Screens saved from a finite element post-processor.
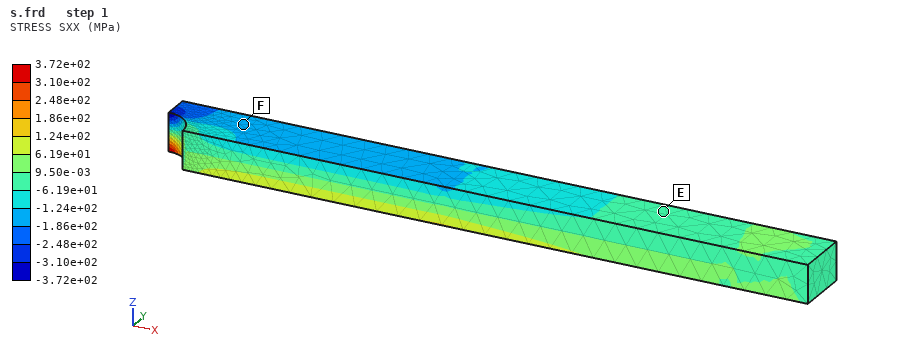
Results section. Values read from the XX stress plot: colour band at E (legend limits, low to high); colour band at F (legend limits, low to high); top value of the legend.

-6.19e+01 to 9.50e-03 MPa
-1.86e+02 to -1.24e+02 MPa
3.72e+02 MPa
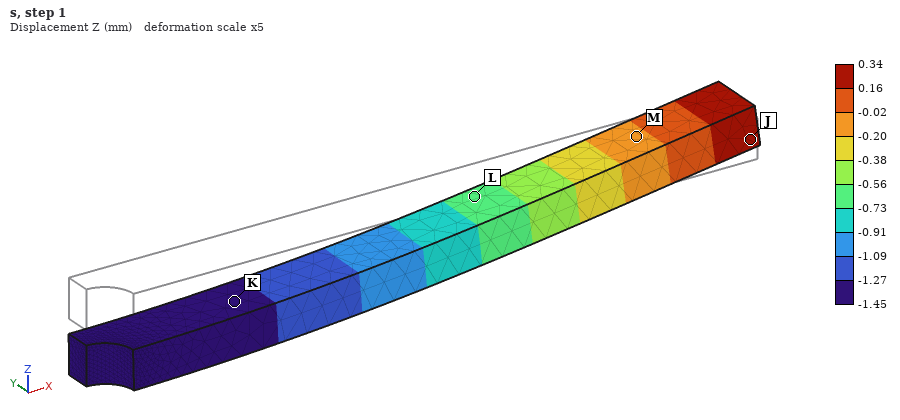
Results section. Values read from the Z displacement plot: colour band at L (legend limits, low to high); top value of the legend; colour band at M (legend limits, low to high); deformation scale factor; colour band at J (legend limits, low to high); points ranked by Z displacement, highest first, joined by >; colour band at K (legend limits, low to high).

-0.73 to -0.56 mm
0.34 mm
-0.20 to -0.02 mm
5
0.16 to 0.34 mm
J > M > L > K
-1.45 to -1.27 mm
